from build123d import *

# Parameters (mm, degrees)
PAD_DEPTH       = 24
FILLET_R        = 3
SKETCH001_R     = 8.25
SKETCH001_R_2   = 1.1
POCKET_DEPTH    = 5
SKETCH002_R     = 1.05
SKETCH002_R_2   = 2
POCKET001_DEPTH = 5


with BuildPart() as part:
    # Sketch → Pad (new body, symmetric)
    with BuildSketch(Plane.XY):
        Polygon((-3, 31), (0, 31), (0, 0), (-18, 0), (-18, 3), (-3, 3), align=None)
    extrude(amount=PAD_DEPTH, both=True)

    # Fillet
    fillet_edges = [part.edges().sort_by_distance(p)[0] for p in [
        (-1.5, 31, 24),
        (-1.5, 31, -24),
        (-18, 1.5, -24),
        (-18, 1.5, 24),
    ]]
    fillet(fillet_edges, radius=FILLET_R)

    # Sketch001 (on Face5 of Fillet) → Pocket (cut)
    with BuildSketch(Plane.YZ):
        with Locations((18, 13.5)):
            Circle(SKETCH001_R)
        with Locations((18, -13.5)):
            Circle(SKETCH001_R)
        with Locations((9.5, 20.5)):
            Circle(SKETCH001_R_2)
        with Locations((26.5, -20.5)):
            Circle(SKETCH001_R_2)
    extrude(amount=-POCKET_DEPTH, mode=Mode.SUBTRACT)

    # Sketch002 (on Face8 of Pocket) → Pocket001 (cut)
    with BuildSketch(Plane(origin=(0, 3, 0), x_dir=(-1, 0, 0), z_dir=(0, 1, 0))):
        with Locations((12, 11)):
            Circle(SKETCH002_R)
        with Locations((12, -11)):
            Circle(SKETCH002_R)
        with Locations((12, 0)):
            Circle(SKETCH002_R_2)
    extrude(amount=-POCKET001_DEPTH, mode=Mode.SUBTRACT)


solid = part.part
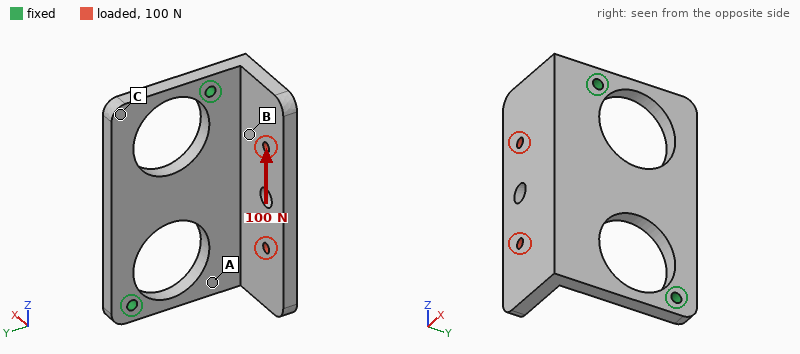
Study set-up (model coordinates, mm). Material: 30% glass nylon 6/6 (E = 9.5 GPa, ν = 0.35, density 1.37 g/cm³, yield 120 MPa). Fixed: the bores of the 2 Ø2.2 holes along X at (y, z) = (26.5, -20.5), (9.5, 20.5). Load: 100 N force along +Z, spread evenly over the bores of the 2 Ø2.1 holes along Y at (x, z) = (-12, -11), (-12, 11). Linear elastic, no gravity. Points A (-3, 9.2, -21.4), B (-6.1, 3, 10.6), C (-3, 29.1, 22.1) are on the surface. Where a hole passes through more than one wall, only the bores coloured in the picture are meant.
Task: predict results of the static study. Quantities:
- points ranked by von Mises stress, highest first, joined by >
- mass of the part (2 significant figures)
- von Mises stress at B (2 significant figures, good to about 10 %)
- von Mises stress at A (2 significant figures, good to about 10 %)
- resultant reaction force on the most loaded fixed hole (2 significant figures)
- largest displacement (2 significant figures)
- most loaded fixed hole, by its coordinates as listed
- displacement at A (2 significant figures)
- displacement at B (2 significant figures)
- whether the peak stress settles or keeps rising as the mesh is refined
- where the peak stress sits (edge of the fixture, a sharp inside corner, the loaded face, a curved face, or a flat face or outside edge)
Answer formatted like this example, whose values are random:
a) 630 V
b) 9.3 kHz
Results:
a) A > B > C
b) 7.2 g
c) 5.6 MPa
d) 9.4 MPa
e) 90 N
f) 0.45 mm
g) (9.5, 20.5)
h) 0.23 mm
i) 0.091 mm
j) keeps rising
k) edge of the fixture
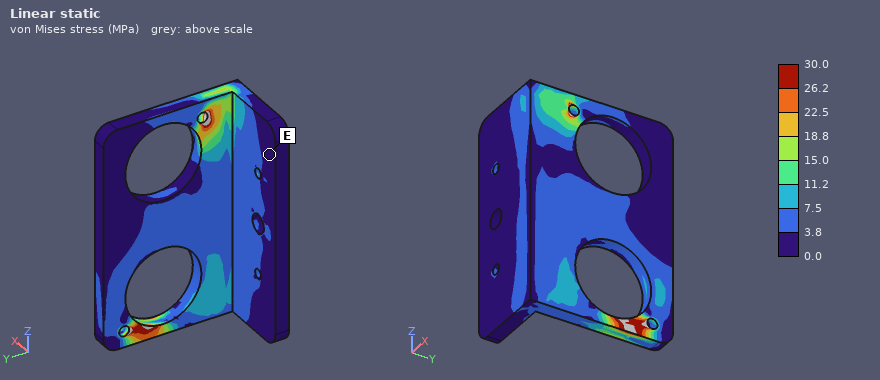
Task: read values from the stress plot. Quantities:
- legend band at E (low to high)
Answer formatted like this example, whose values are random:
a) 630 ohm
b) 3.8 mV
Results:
a) 0.0 to 3.8 MPa
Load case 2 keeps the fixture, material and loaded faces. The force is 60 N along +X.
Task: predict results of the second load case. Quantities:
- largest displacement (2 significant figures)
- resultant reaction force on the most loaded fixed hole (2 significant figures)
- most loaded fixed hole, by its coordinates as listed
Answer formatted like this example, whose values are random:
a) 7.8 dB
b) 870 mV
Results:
a) 0.61 mm
b) 42 N
c) (9.5, 20.5)
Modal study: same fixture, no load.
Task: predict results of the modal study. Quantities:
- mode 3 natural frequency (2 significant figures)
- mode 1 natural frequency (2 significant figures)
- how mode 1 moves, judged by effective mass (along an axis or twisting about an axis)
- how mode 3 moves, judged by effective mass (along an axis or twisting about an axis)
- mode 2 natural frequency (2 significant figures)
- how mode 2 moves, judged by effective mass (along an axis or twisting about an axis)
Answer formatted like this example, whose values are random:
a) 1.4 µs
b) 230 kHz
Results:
a) 2600 Hz
b) 910 Hz
c) along X
d) along Y
e) 2000 Hz
f) along X
